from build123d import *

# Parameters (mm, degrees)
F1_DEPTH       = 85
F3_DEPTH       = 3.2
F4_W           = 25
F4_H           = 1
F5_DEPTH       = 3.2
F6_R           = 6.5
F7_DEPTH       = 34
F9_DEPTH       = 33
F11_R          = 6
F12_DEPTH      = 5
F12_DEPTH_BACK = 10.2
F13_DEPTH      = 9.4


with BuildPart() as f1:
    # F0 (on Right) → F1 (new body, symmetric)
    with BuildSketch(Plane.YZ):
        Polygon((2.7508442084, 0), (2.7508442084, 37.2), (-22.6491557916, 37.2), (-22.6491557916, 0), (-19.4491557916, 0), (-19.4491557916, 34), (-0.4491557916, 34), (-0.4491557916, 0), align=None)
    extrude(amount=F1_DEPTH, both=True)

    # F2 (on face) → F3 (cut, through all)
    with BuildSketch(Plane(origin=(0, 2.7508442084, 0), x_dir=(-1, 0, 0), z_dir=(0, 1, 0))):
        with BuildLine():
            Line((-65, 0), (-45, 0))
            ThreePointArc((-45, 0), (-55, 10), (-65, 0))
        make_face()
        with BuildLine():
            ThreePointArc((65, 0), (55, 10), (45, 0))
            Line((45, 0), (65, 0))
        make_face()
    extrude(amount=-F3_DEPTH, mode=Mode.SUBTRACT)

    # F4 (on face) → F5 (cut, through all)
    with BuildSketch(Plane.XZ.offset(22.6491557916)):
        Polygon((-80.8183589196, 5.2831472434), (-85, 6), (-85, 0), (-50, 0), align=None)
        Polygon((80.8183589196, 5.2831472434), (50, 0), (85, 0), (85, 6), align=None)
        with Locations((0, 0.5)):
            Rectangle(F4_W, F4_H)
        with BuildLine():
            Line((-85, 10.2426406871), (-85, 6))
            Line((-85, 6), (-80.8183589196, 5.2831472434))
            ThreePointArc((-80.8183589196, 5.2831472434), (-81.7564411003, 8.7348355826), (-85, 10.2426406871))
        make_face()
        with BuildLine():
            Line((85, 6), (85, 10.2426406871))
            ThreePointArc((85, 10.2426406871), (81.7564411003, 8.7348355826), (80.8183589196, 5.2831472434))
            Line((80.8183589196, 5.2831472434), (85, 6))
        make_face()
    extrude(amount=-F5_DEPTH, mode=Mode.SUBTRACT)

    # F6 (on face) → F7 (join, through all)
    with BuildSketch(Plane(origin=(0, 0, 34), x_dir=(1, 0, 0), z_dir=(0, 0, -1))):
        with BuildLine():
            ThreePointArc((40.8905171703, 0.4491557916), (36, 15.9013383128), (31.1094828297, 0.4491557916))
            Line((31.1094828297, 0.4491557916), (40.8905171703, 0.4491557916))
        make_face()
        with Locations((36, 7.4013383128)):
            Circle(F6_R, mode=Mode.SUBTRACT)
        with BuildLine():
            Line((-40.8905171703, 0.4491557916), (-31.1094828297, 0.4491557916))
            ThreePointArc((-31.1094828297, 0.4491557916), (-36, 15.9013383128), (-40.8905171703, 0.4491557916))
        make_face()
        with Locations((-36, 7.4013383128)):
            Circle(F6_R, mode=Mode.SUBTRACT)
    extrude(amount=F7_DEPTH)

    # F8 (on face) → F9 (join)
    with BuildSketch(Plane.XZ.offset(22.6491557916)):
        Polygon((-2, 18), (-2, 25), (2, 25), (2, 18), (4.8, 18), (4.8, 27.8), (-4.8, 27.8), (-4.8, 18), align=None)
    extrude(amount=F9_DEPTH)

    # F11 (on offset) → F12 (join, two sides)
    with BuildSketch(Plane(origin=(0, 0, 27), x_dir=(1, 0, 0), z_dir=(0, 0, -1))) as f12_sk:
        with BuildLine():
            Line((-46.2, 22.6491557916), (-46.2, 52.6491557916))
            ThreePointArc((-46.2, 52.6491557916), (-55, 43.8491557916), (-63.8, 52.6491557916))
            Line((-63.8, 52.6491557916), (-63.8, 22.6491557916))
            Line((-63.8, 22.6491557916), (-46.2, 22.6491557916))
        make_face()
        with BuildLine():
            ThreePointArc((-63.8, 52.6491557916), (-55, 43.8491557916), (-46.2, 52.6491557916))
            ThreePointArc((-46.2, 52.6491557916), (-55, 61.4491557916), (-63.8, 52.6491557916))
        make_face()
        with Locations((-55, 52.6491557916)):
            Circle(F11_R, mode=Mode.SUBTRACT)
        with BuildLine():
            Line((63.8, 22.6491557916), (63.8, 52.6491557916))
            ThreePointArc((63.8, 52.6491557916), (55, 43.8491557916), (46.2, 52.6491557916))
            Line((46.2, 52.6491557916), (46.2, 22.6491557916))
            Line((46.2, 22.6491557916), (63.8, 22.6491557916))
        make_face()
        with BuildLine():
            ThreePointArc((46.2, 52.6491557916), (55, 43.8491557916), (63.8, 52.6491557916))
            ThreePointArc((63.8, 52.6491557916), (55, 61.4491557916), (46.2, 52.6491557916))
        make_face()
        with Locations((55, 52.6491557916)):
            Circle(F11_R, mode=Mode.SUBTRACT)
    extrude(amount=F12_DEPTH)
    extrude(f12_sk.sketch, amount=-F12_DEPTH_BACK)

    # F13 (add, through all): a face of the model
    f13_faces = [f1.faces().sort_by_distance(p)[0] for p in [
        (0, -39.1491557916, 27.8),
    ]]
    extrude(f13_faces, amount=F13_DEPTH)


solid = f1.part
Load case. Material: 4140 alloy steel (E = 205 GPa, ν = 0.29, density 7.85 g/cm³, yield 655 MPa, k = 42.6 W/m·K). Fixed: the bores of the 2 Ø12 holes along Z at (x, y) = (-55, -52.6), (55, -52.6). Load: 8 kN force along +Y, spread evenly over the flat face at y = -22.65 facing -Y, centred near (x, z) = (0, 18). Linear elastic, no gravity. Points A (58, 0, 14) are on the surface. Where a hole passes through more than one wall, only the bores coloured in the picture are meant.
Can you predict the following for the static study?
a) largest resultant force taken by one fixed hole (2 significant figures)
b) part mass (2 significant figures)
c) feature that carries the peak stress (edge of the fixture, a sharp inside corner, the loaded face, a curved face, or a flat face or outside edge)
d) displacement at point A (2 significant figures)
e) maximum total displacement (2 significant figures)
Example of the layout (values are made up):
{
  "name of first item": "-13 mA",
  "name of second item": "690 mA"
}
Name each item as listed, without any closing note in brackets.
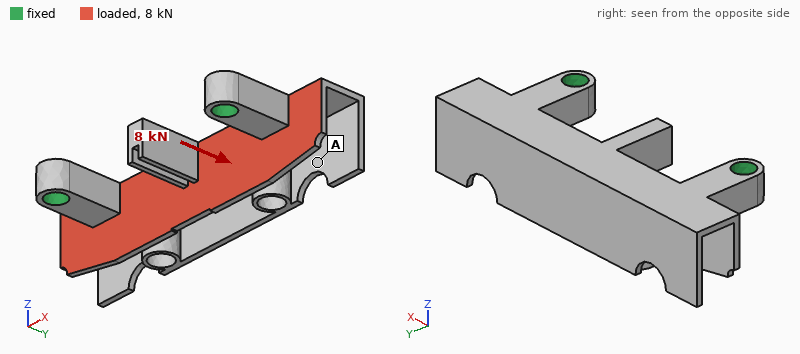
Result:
{
  "largest resultant force taken by one fixed hole": "4.2 kN",
  "part mass": "600 g",
  "feature that carries the peak stress": "a flat face or outside edge",
  "displacement at point A": "0.15 mm",
  "maximum total displacement": "0.48 mm"
}
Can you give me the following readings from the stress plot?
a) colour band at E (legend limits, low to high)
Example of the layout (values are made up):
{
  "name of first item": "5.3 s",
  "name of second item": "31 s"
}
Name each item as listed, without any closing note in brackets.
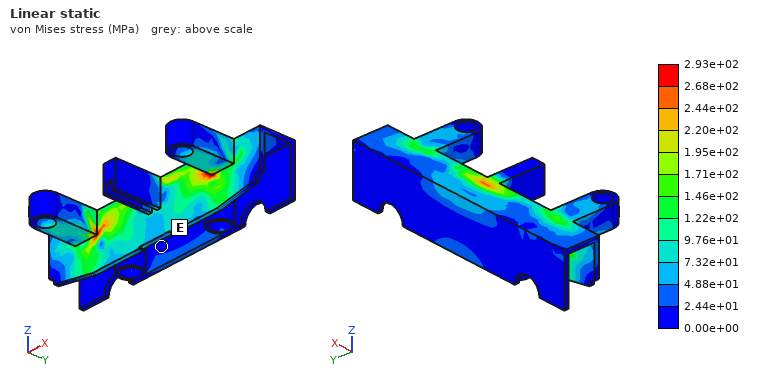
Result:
{
  "colour band at E": "0.00e+00 to 2.44e+01 MPa"
}
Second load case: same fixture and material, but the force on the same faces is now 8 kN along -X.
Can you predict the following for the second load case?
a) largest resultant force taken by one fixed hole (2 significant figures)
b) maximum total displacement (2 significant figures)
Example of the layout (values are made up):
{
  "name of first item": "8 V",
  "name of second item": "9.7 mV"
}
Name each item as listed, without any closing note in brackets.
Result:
{
  "largest resultant force taken by one fixed hole": "4.1 kN",
  "maximum total displacement": "38 µm"
}
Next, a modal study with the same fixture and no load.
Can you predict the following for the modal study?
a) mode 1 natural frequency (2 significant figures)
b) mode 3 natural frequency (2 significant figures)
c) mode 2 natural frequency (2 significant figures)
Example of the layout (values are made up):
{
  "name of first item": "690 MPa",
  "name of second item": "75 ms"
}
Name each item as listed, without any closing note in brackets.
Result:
{
  "mode 1 natural frequency": "980 Hz",
  "mode 3 natural frequency": "1900 Hz",
  "mode 2 natural frequency": "1500 Hz"
}
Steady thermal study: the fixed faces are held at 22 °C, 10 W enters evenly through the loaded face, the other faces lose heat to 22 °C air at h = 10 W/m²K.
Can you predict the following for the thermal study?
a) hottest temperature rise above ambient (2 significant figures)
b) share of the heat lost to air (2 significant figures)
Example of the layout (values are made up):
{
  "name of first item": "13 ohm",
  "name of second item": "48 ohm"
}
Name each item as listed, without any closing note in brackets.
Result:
{
  "hottest temperature rise above ambient": "17 K",
  "share of the heat lost to air": "35 %"
}
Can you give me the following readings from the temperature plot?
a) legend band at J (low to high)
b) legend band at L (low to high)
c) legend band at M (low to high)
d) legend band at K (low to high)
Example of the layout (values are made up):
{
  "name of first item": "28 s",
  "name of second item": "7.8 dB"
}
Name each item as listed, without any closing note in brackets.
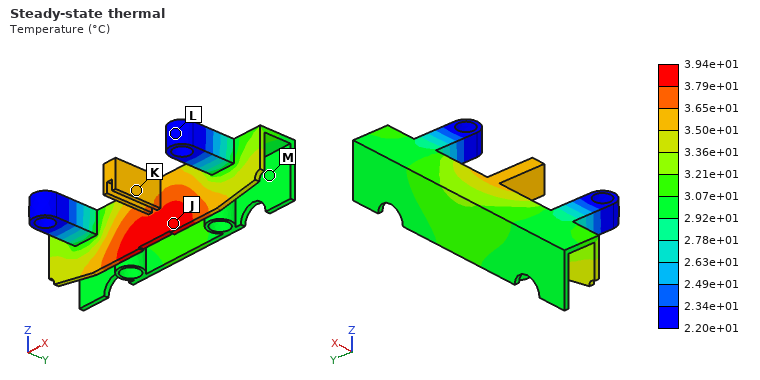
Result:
{
  "legend band at J": "3.79e+01 to 3.94e+01 °C",
  "legend band at L": "2.20e+01 to 2.34e+01 °C",
  "legend band at M": "2.92e+01 to 3.07e+01 °C",
  "legend band at K": "3.50e+01 to 3.65e+01 °C"
}
